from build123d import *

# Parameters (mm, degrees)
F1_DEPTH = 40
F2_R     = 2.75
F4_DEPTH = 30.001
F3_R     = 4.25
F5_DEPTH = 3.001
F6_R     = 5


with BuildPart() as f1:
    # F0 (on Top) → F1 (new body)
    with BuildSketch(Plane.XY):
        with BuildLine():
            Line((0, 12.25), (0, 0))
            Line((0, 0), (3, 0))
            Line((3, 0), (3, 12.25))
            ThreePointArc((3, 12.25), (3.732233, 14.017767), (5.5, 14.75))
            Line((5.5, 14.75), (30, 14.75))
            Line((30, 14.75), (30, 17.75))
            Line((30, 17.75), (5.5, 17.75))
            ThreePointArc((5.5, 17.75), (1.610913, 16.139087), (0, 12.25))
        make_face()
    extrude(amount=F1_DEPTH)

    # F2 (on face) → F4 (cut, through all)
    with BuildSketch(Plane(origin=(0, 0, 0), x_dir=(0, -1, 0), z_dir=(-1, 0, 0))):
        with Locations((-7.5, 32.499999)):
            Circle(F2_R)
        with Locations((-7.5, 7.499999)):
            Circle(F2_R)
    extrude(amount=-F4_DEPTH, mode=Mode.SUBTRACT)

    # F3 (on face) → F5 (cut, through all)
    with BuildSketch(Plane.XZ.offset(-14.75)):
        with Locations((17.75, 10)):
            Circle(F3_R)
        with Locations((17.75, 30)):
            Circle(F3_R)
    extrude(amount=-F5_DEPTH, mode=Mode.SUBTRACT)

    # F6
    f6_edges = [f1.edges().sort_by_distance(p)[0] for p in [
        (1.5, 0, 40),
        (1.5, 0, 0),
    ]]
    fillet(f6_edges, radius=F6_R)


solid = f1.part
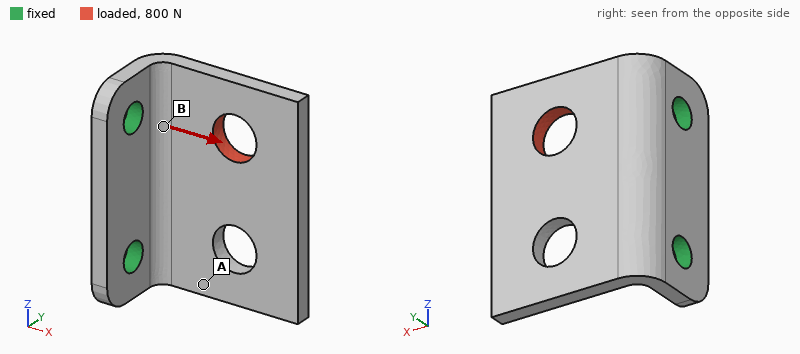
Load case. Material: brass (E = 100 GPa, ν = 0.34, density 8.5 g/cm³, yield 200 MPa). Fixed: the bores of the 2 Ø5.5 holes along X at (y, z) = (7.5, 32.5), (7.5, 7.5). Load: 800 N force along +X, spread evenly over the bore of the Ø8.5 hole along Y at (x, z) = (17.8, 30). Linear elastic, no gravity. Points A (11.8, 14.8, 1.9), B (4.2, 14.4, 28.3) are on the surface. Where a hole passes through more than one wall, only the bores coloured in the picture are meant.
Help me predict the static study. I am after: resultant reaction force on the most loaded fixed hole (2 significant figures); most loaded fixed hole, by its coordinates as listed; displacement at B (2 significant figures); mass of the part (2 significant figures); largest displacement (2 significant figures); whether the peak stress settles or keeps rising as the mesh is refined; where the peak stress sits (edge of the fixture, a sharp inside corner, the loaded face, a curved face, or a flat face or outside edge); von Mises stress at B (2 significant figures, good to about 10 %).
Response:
700 N
(7.5, 32.5)
0.016 mm
40 g
0.10 mm
keeps rising
edge of the fixture
45 MPa
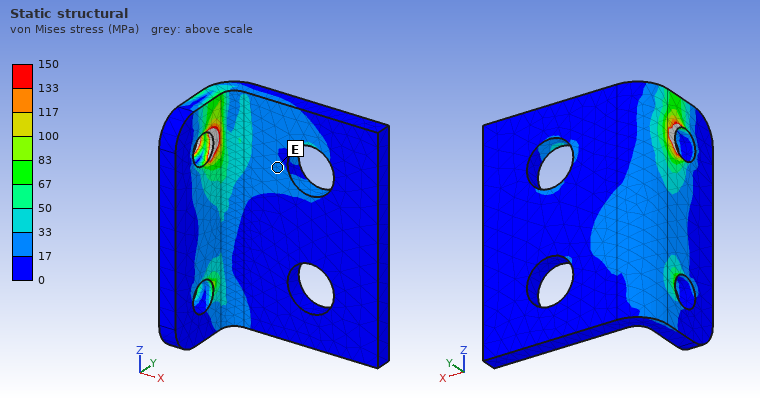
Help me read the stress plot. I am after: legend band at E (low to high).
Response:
17 to 33 MPa
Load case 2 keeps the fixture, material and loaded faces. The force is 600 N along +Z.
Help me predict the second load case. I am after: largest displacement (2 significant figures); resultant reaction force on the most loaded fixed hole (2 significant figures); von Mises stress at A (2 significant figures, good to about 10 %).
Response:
38 µm
490 N
17 MPa
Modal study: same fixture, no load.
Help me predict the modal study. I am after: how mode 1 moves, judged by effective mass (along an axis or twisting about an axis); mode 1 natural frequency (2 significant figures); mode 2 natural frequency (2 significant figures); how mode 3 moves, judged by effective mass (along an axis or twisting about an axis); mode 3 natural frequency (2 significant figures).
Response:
along Y
1600 Hz
3200 Hz
along Z
6000 Hz
